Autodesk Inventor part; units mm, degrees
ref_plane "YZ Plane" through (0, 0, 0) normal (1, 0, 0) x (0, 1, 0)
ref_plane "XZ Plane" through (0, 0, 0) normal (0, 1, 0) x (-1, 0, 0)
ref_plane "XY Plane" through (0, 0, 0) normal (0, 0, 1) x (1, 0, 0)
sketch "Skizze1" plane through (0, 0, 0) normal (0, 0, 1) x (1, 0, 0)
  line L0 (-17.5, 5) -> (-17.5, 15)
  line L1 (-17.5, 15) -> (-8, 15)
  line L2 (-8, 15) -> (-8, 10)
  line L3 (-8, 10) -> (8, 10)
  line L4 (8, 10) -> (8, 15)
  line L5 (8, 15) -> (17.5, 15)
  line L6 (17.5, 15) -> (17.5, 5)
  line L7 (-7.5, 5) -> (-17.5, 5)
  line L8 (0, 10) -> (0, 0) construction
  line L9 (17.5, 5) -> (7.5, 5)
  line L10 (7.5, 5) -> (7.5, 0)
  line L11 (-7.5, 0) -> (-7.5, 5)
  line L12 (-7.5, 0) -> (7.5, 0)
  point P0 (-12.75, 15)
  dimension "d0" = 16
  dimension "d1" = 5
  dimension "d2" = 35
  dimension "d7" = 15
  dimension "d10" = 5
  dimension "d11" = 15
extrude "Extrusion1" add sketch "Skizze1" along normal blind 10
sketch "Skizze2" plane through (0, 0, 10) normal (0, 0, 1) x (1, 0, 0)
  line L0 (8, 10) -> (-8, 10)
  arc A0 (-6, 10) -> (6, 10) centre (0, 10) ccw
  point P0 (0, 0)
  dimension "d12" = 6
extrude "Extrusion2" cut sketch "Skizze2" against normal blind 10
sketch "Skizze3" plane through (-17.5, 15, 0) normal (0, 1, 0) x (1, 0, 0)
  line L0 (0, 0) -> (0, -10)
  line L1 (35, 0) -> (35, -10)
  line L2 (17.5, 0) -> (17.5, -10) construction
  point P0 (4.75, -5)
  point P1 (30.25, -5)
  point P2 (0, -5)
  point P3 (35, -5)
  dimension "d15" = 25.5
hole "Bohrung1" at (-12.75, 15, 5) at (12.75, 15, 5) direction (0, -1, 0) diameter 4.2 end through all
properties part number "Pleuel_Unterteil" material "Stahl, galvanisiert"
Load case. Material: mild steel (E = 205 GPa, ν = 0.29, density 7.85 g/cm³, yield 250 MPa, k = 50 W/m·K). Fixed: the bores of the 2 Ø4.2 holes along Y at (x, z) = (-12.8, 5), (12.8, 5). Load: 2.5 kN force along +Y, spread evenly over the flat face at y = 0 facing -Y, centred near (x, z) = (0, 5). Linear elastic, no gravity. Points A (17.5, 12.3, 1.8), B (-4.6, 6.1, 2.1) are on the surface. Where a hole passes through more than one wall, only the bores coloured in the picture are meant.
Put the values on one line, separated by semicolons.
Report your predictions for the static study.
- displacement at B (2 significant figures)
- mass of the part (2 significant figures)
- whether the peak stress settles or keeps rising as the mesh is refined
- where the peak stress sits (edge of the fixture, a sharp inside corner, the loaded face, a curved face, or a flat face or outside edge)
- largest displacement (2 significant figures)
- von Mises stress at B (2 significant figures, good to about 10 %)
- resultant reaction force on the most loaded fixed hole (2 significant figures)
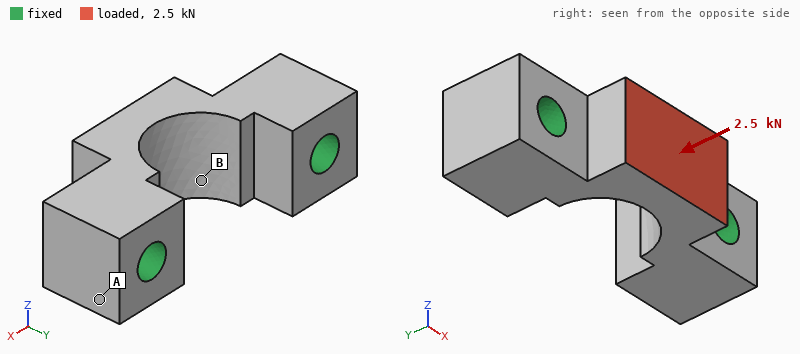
2.4 µm; 20 g; keeps rising; edge of the fixture; 3.6 µm; 36 MPa; 1.5 kN
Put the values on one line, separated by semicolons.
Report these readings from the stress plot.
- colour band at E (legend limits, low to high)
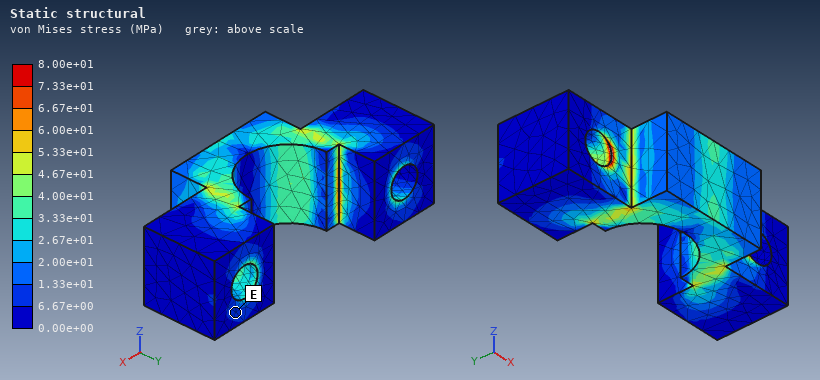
6.67e+00 to 1.33e+01 MPa
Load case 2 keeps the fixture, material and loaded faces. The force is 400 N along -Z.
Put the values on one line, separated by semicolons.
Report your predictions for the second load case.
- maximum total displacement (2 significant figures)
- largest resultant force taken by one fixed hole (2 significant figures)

3.2 µm; 200 N
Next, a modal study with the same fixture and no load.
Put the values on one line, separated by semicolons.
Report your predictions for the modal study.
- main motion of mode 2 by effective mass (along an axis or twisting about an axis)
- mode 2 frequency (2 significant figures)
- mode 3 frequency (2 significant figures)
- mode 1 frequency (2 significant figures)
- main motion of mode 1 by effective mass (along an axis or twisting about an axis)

along Y; 57 kHz; 61 kHz; 31 kHz; along Z
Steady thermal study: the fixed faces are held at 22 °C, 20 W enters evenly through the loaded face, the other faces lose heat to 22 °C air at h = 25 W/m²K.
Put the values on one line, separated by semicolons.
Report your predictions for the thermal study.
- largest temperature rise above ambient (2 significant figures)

50 K
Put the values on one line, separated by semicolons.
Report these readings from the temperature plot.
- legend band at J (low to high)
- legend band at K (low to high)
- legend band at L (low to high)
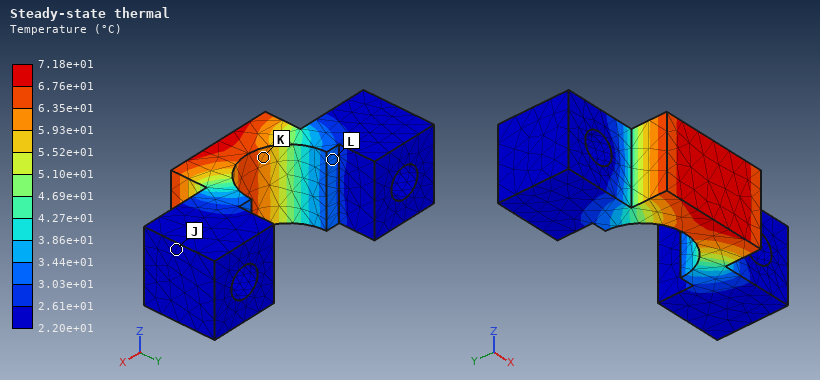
2.20e+01 to 2.61e+01 °C; 5.93e+01 to 6.35e+01 °C; 3.03e+01 to 3.44e+01 °C
